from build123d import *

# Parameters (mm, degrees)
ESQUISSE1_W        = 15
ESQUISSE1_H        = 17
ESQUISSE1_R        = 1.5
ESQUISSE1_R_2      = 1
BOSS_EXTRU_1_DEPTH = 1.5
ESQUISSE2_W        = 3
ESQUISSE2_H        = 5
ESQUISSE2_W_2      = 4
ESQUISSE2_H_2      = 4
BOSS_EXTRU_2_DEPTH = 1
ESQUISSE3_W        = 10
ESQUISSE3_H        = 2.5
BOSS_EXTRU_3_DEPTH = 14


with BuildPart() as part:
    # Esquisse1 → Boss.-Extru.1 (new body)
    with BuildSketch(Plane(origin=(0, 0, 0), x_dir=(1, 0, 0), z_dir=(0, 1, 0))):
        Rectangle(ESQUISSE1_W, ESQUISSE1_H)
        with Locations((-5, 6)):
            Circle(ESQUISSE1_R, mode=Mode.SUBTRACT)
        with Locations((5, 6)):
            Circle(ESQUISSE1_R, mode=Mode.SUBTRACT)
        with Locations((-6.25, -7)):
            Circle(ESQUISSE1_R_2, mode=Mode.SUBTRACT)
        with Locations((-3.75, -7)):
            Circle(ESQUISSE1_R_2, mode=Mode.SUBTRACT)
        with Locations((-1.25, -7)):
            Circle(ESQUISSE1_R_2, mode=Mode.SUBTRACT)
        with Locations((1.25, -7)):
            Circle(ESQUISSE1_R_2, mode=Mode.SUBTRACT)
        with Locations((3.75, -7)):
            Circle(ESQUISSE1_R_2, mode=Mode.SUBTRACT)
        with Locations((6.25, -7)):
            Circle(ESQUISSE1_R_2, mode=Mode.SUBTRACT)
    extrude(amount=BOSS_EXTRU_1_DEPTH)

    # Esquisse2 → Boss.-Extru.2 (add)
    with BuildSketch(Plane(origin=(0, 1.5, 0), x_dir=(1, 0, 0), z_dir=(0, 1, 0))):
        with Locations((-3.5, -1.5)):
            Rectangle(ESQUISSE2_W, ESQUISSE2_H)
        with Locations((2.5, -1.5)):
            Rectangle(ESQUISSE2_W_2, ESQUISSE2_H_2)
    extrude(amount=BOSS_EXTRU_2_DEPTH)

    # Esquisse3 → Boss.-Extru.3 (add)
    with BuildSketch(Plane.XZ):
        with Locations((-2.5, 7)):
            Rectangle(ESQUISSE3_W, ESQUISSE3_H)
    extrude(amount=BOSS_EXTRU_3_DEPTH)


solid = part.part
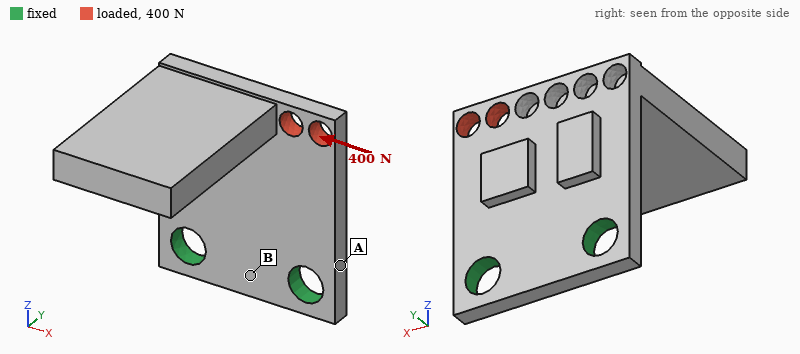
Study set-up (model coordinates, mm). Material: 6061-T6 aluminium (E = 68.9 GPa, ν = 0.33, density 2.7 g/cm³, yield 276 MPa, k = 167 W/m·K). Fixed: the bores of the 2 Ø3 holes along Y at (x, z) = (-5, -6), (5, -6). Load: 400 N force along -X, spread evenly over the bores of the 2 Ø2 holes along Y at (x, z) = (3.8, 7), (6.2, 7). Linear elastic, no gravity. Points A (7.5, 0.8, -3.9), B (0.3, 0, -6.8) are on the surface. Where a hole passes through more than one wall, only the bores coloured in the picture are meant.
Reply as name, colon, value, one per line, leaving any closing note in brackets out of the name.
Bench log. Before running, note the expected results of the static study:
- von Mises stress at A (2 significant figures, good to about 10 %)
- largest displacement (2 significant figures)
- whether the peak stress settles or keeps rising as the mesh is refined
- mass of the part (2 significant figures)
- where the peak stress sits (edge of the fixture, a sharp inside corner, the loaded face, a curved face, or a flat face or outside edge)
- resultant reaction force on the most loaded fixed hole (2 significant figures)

von Mises stress at A: 70 MPa
largest displacement: 33 µm
whether the peak stress settles or keeps rising as the mesh is refined: keeps rising
mass of the part: 1.9 g
where the peak stress sits: a sharp inside corner
resultant reaction force on the most loaded fixed hole: 490 N
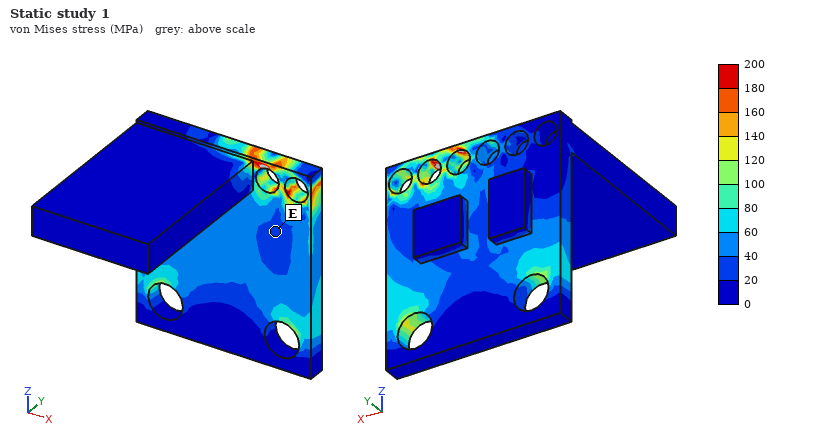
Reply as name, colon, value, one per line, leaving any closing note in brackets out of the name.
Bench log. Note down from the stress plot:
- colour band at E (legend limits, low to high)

colour band at E: 20 to 40 MPa
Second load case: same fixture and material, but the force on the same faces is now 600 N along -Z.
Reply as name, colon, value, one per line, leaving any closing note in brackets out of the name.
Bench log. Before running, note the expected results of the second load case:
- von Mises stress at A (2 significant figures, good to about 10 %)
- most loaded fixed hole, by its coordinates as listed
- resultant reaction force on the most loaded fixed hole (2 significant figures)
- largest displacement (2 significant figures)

von Mises stress at A: 58 MPa
most loaded fixed hole, by its coordinates as listed: (5, -6)
resultant reaction force on the most loaded fixed hole: 580 N
largest displacement: 25 µm
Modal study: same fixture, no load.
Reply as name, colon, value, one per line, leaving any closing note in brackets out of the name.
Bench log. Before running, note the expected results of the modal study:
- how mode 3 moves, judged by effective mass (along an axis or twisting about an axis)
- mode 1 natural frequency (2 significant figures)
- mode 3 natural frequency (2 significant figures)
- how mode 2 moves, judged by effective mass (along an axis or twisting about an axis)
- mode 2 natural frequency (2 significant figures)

how mode 3 moves, judged by effective mass: along Y
mode 1 natural frequency: 2300 Hz
mode 3 natural frequency: 6600 Hz
how mode 2 moves, judged by effective mass: along X
mode 2 natural frequency: 4400 Hz
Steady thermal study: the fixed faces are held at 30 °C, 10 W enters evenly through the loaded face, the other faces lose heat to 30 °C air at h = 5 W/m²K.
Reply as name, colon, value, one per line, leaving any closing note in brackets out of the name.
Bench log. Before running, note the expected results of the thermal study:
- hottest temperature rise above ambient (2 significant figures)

hottest temperature rise above ambient: 65 K
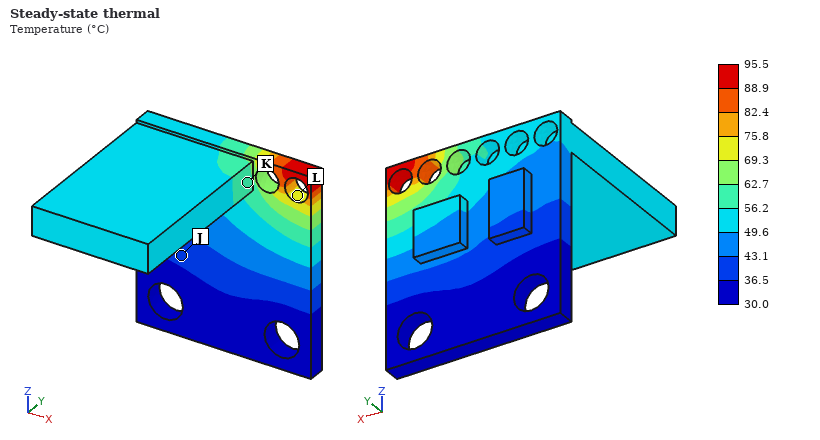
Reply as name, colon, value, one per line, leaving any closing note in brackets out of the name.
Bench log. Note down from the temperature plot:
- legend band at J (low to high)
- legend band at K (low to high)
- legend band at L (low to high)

legend band at J: 36.5 to 43.1 °C
legend band at K: 56.2 to 62.7 °C
legend band at L: 69.3 to 75.8 °C
